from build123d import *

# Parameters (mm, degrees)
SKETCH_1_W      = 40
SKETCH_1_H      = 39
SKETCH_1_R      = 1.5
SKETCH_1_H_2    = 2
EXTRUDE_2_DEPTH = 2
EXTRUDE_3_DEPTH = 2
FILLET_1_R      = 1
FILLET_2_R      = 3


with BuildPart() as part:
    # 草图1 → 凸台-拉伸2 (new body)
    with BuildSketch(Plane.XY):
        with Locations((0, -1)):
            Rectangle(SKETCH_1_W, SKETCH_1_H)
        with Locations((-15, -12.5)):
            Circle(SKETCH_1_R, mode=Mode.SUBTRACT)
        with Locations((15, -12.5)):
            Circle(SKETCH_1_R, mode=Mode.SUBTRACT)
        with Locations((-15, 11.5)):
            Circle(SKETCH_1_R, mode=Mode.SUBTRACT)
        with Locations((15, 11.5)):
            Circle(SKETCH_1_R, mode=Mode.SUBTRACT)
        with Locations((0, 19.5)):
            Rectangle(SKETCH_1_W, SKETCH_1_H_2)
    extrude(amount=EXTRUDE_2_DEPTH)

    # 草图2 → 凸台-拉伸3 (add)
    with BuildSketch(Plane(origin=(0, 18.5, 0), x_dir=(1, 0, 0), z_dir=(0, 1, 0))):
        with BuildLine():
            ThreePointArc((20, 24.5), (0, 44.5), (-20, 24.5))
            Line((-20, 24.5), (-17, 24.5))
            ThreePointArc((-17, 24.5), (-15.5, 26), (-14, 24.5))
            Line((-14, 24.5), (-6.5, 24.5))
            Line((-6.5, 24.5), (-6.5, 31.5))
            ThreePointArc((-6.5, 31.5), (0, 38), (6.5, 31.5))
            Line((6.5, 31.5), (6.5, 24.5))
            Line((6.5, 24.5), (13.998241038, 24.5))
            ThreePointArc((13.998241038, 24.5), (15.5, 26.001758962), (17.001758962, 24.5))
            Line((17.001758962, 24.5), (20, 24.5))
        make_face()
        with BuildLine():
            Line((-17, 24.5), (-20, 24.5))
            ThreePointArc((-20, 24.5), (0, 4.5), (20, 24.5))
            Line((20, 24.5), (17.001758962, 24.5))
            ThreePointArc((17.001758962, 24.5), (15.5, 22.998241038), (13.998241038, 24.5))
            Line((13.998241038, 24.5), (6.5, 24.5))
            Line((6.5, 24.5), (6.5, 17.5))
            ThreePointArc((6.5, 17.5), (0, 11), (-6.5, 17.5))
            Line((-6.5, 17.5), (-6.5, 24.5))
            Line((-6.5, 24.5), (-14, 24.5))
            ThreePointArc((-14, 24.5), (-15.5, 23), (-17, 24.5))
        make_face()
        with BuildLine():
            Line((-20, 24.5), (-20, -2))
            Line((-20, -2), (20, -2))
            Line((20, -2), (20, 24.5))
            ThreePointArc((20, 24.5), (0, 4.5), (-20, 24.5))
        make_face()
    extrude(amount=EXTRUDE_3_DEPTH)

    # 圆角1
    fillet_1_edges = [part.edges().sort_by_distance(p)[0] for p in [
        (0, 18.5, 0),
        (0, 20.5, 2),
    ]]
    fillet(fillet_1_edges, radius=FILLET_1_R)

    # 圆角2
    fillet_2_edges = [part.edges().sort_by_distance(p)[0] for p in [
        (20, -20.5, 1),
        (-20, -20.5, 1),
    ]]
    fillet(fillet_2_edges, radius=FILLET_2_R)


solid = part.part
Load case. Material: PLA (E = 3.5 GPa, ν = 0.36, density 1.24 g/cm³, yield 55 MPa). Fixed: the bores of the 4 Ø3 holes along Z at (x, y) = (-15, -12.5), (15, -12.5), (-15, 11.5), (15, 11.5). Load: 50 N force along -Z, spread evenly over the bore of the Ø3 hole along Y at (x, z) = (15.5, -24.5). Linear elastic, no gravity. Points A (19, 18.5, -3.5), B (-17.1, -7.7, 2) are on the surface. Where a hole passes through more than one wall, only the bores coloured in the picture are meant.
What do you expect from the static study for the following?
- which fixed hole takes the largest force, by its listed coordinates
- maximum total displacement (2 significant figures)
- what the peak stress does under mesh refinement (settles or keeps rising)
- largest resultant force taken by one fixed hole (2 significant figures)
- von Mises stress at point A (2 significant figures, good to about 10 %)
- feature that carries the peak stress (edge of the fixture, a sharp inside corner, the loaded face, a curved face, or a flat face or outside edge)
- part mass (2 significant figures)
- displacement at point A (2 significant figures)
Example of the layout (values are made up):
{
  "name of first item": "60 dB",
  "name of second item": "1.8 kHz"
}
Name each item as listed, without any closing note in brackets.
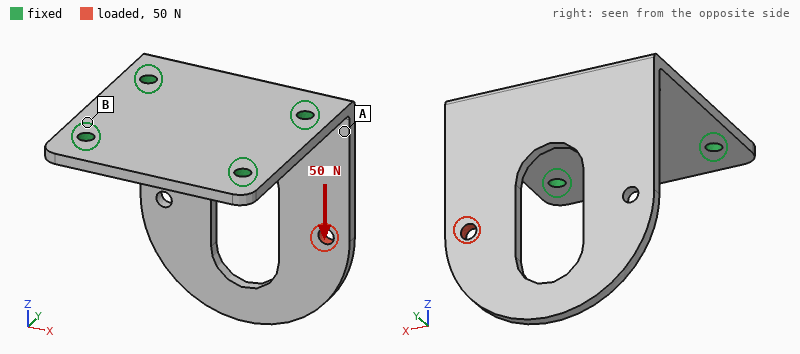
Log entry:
{
  "which fixed hole takes the largest force, by its listed coordinates": "(15, 11.5)",
  "maximum total displacement": "0.88 mm",
  "what the peak stress does under mesh refinement": "keeps rising",
  "largest resultant force taken by one fixed hole": "53 N",
  "von Mises stress at point A": "7.5 MPa",
  "feature that carries the peak stress": "edge of the fixture",
  "part mass": "7.2 g",
  "displacement at point A": "0.23 mm"
}
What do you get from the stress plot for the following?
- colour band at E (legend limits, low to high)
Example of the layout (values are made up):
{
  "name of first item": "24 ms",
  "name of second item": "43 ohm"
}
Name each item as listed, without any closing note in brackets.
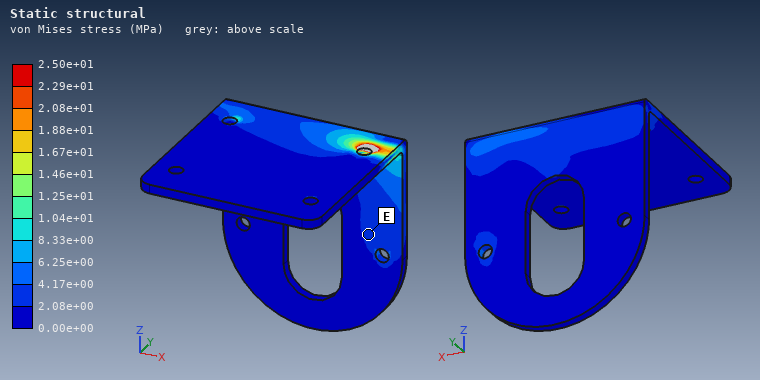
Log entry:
{
  "colour band at E": "2.08e+00 to 4.17e+00 MPa"
}
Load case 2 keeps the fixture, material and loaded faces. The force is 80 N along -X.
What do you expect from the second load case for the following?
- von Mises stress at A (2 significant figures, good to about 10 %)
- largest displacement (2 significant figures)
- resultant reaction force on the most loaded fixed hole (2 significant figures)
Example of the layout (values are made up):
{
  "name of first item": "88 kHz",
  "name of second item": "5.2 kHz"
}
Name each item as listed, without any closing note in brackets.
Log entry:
{
  "von Mises stress at A": "15 MPa",
  "largest displacement": "0.78 mm",
  "resultant reaction force on the most loaded fixed hole": "82 N"
}
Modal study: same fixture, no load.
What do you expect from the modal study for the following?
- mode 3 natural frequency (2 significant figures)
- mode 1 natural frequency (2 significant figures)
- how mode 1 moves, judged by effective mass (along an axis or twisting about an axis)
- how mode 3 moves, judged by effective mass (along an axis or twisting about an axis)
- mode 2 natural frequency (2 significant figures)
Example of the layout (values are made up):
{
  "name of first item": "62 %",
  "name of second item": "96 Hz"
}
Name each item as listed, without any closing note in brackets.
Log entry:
{
  "mode 3 natural frequency": "1300 Hz",
  "mode 1 natural frequency": "270 Hz",
  "how mode 1 moves, judged by effective mass": "along Y",
  "how mode 3 moves, judged by effective mass": "along X",
  "mode 2 natural frequency": "720 Hz"
}
